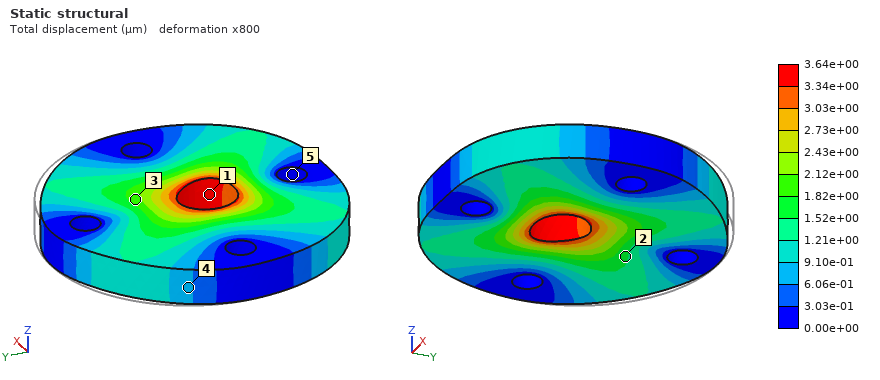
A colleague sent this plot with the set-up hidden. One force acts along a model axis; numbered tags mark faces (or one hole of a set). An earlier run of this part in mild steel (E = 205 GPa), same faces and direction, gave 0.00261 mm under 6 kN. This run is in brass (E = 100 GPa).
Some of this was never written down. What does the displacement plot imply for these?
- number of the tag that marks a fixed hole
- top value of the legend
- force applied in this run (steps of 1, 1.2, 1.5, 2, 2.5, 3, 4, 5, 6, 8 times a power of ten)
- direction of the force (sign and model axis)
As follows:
5
3.64e+00 µm
4 kN
-Y
